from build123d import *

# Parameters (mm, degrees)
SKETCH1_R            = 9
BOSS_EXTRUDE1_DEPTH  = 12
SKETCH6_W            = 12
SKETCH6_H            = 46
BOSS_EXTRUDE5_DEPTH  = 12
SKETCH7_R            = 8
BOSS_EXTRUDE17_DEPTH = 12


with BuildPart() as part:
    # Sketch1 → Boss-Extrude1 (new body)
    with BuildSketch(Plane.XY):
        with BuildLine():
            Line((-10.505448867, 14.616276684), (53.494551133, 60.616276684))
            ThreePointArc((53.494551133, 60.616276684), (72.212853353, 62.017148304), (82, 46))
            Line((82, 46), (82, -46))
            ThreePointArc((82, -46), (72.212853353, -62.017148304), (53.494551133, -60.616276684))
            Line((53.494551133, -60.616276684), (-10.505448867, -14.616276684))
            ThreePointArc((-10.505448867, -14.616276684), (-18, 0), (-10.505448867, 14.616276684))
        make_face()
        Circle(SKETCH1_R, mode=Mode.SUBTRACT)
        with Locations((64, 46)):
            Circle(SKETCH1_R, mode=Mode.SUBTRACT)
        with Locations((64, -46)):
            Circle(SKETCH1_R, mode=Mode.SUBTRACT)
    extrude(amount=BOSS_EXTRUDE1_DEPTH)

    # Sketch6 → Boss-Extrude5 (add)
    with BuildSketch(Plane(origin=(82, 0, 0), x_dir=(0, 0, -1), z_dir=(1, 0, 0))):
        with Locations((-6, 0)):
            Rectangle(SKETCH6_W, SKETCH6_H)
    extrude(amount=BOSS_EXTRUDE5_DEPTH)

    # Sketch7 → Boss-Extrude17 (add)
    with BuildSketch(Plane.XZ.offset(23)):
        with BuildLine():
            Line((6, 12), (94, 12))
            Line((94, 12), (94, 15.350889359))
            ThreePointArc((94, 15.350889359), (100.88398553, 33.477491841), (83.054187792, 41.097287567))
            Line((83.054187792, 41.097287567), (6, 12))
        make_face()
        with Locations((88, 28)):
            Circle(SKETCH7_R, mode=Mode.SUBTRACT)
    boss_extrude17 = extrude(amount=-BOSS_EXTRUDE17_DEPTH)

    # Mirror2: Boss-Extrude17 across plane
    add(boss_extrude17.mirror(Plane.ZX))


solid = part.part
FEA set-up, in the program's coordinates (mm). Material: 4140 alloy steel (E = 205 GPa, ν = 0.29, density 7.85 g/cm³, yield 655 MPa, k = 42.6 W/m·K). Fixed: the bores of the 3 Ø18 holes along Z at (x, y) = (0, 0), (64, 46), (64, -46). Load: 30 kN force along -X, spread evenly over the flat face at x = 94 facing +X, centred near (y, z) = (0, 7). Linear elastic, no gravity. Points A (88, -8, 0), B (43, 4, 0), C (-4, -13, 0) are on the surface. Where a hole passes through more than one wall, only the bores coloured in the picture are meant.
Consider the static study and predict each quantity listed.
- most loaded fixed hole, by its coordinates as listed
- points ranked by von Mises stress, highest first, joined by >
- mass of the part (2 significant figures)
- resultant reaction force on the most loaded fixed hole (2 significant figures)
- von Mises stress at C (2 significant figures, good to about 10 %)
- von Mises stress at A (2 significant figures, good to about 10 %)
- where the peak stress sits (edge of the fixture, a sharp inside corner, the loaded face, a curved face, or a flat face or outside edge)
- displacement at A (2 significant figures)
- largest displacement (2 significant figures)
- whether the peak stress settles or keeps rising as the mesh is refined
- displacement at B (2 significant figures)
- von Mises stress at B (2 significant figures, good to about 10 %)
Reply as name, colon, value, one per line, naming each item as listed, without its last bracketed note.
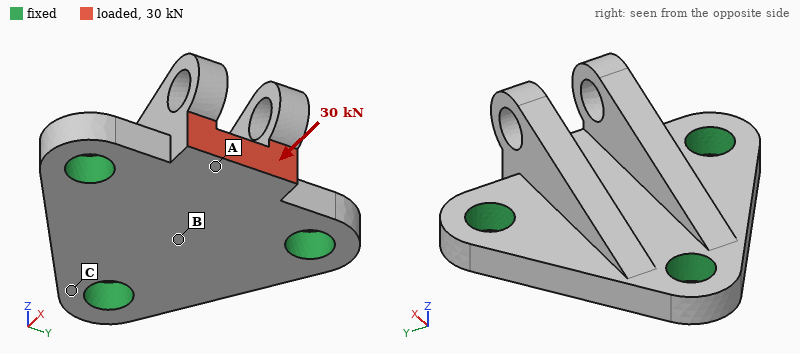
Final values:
most loaded fixed hole, by its coordinates as listed: (0, 0)
points ranked by von Mises stress, highest first, joined by >: A > B > C
mass of the part: 1.0 kg
resultant reaction force on the most loaded fixed hole: 11 kN
von Mises stress at C: 12 MPa
von Mises stress at A: 42 MPa
where the peak stress sits: a sharp inside corner
displacement at A: 13 µm
largest displacement: 15 µm
whether the peak stress settles or keeps rising as the mesh is refined: keeps rising
displacement at B: 4.6 µm
von Mises stress at B: 30 MPa
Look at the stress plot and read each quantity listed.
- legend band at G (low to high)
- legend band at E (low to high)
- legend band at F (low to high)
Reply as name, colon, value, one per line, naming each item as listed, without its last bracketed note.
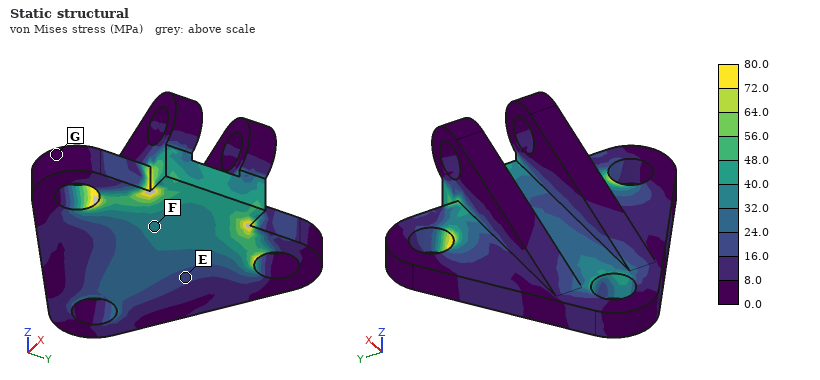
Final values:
legend band at G: 0.0 to 8.0 MPa
legend band at E: 16.0 to 24.0 MPa
legend band at F: 32.0 to 40.0 MPa
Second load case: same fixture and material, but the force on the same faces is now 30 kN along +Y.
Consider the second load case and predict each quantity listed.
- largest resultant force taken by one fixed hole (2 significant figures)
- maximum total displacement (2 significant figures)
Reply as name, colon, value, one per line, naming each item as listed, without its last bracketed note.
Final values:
largest resultant force taken by one fixed hole: 18 kN
maximum total displacement: 29 µm
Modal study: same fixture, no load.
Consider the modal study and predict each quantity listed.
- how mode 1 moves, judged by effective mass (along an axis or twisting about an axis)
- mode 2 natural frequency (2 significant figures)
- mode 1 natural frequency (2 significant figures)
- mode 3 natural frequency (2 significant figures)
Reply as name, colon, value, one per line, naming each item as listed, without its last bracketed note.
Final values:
how mode 1 moves, judged by effective mass: along Z
mode 2 natural frequency: 8100 Hz
mode 1 natural frequency: 5100 Hz
mode 3 natural frequency: 8300 Hz
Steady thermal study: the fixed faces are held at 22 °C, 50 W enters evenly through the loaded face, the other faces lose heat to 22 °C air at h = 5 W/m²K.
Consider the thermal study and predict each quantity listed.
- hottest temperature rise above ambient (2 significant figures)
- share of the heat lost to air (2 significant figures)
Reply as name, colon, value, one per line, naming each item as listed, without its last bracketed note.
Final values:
hottest temperature rise above ambient: 60 K
share of the heat lost to air: 4.1 %
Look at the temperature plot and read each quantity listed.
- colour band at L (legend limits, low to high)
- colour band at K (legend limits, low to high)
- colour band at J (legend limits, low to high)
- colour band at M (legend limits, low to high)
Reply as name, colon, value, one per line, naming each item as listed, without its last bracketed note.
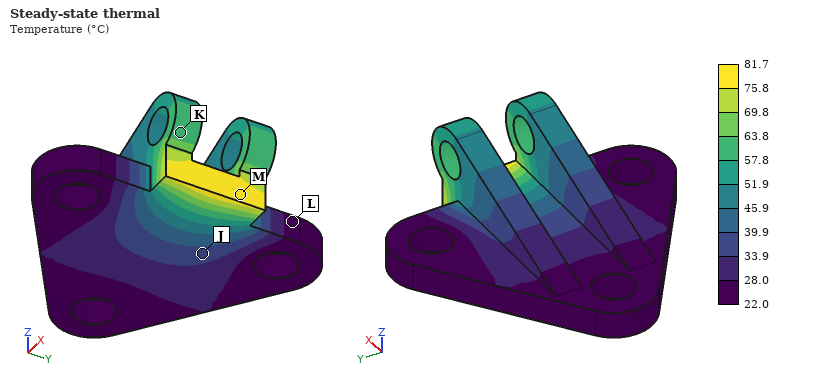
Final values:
colour band at L: 22.0 to 28.0 °C
colour band at K: 57.8 to 63.8 °C
colour band at J: 33.9 to 39.9 °C
colour band at M: 75.8 to 81.7 °C
